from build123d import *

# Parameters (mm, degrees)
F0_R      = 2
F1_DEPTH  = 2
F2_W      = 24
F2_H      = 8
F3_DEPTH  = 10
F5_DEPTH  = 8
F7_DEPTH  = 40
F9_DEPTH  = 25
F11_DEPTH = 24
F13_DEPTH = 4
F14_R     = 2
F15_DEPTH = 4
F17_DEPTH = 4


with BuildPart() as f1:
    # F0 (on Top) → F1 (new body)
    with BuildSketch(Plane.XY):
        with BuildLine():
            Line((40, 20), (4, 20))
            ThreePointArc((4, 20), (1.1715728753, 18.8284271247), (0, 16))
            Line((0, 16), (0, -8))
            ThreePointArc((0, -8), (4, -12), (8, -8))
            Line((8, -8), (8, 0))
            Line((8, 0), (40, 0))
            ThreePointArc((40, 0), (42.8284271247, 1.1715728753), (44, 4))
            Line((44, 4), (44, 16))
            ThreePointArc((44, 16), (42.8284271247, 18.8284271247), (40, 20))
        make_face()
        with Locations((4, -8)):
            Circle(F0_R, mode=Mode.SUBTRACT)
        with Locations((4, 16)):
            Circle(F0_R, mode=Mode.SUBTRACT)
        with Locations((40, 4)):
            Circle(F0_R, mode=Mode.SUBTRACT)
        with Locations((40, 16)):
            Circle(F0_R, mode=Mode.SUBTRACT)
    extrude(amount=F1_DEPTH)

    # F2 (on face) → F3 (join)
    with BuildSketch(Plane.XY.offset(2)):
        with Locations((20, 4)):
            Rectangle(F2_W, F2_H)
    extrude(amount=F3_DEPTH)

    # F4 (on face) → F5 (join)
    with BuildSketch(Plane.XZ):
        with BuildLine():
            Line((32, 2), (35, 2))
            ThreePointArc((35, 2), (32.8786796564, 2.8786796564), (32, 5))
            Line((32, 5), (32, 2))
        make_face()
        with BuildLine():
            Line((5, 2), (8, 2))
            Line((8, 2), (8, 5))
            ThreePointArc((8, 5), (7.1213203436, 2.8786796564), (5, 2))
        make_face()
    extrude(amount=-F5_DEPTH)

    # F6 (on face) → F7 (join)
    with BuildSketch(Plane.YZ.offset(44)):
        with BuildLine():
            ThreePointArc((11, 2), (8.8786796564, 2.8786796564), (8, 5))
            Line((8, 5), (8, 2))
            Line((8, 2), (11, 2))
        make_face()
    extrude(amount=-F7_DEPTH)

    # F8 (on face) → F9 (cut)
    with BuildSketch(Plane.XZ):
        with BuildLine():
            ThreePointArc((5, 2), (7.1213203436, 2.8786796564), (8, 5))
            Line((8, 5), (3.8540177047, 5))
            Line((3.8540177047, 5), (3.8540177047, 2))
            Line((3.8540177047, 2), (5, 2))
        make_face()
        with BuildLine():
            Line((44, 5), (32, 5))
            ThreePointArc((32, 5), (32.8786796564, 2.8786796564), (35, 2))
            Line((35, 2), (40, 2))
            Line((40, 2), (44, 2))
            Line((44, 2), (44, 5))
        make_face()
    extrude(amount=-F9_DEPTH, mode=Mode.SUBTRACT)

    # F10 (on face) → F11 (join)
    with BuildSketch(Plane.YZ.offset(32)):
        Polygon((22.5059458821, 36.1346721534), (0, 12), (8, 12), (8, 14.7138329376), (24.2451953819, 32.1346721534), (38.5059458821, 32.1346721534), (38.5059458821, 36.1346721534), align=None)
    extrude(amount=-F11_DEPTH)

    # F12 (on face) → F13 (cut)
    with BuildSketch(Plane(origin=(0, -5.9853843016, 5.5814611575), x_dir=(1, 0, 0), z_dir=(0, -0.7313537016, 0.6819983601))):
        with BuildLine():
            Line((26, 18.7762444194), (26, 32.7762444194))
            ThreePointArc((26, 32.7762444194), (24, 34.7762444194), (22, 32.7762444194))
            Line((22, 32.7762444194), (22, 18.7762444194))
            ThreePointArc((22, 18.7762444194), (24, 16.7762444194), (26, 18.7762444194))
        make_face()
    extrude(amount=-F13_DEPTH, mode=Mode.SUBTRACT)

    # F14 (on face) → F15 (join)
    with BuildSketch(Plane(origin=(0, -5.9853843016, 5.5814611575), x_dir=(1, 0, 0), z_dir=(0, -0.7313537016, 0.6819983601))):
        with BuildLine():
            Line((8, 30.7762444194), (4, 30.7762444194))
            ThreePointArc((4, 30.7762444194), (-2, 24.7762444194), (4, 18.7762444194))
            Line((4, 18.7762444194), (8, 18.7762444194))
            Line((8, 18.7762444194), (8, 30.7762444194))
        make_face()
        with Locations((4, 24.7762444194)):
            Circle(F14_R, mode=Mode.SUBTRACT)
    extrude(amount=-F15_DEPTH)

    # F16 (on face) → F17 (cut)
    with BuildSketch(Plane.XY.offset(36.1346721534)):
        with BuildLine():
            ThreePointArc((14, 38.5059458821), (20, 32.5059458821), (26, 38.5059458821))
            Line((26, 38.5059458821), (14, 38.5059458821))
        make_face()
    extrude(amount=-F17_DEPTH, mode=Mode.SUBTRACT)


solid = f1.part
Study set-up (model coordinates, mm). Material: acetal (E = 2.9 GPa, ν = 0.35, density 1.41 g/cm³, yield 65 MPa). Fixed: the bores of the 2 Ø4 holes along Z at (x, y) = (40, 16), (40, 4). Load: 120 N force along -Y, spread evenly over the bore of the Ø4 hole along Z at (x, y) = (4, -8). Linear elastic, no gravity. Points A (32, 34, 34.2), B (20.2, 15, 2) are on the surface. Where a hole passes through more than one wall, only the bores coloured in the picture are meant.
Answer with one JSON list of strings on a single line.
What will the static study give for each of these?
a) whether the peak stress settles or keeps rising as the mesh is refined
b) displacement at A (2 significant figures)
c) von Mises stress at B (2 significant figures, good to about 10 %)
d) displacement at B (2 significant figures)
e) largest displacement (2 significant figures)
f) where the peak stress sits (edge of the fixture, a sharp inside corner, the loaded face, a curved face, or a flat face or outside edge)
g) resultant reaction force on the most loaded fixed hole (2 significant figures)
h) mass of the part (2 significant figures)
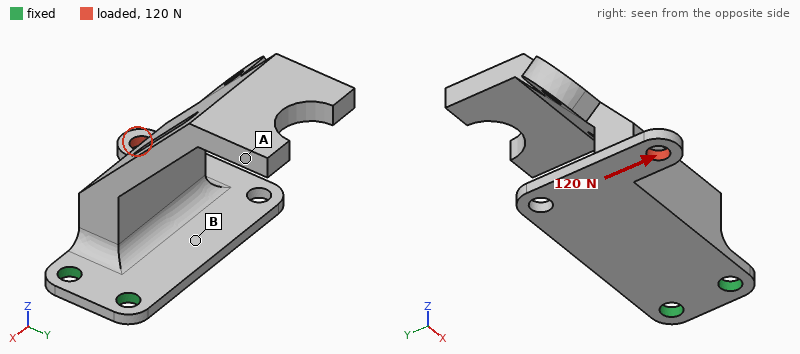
["keeps rising", "0.62 mm", "8.3 MPa", "0.25 mm", "0.76 mm", "edge of the fixture", "310 N", "11 g"]
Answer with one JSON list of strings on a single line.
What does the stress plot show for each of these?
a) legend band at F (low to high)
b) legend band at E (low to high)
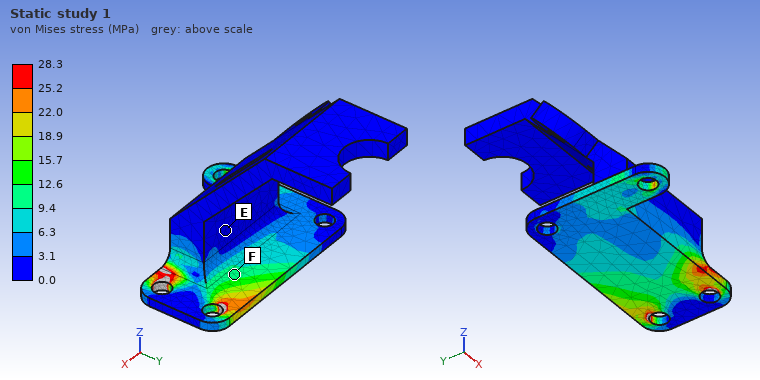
["9.4 to 12.6 MPa", "0.0 to 3.1 MPa"]
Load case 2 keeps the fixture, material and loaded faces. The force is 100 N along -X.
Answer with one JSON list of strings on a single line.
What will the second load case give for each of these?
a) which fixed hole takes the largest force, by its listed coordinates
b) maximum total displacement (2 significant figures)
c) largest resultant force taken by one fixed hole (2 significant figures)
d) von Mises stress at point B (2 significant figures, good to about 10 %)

["(40, 4)", "0.84 mm", "180 N", "4.2 MPa"]
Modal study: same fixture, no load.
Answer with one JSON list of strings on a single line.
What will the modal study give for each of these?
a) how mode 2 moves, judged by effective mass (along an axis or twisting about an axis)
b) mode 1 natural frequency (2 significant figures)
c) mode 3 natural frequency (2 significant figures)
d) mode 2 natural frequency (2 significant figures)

["along Y", "130 Hz", "1000 Hz", "250 Hz"]
